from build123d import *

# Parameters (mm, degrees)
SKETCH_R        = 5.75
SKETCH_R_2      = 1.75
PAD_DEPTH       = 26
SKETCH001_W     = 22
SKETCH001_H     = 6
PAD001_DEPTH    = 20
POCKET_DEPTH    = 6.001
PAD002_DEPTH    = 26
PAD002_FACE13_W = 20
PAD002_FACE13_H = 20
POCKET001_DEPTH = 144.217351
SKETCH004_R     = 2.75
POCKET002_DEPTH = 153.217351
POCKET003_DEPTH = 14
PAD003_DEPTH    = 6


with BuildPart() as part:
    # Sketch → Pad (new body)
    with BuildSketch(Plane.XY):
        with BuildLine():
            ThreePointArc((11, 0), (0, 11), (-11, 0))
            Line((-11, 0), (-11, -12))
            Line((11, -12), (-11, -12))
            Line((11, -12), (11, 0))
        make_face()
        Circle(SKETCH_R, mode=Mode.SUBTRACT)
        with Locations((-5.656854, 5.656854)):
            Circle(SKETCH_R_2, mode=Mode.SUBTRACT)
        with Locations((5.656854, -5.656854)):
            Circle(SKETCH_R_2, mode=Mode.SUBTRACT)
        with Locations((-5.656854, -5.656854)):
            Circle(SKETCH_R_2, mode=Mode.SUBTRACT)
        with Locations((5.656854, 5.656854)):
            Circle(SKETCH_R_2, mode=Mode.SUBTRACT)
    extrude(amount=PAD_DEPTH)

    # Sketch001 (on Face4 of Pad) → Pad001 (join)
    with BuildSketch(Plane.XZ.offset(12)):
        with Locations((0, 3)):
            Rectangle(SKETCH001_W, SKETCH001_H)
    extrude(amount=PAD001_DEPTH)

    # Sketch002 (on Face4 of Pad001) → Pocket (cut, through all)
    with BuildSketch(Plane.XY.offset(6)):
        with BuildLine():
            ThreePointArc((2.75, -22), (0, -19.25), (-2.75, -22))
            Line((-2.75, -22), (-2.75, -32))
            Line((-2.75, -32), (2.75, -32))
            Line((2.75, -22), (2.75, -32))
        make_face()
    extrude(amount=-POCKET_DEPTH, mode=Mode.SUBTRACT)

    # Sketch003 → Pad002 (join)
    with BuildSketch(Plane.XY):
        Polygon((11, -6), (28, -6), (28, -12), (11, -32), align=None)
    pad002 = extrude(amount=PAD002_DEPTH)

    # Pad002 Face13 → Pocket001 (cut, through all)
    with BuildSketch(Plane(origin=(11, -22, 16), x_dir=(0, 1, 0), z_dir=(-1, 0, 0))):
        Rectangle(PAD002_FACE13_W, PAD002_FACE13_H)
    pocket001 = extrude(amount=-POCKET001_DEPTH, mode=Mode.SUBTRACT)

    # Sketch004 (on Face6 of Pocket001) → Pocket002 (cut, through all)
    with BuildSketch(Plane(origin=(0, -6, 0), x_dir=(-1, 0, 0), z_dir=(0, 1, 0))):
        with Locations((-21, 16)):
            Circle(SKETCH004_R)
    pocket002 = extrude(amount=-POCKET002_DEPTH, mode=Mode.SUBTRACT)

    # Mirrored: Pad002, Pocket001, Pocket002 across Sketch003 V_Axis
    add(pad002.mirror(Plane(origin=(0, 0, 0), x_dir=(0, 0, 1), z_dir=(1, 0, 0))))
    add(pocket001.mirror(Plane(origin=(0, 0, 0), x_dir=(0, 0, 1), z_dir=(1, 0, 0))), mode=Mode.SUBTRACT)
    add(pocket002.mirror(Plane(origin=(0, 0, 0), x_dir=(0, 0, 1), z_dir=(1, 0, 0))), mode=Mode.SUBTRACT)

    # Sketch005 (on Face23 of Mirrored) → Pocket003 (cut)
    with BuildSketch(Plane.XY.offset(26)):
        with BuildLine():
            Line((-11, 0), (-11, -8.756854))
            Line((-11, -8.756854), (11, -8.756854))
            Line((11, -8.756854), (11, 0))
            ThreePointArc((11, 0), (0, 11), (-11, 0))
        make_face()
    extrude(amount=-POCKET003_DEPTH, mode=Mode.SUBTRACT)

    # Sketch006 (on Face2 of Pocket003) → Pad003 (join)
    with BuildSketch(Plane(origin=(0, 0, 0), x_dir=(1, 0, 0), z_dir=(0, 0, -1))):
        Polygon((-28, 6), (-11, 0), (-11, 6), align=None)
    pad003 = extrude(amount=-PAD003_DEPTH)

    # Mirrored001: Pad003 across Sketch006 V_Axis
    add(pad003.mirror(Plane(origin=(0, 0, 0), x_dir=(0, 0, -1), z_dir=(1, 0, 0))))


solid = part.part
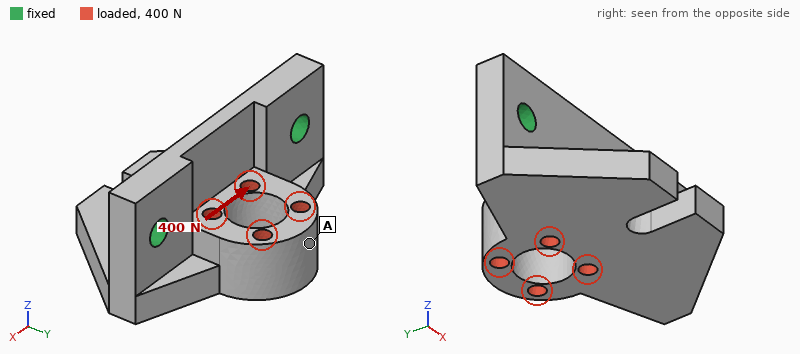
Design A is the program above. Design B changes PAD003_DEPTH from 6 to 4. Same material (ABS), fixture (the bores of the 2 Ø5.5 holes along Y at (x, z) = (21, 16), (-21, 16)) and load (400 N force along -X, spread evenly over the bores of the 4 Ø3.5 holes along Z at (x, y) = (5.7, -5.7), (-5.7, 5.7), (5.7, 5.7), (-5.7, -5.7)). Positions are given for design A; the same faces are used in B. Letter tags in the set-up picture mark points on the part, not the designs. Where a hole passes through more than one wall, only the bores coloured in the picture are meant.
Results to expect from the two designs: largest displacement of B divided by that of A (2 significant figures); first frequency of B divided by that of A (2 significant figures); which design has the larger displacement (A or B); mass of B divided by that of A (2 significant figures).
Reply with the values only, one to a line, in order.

1.1
1.00
B
0.99
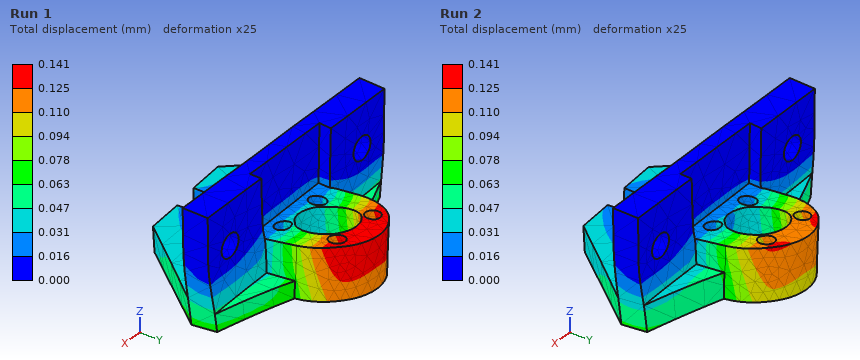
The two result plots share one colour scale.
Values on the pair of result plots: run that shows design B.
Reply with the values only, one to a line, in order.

Run 1
